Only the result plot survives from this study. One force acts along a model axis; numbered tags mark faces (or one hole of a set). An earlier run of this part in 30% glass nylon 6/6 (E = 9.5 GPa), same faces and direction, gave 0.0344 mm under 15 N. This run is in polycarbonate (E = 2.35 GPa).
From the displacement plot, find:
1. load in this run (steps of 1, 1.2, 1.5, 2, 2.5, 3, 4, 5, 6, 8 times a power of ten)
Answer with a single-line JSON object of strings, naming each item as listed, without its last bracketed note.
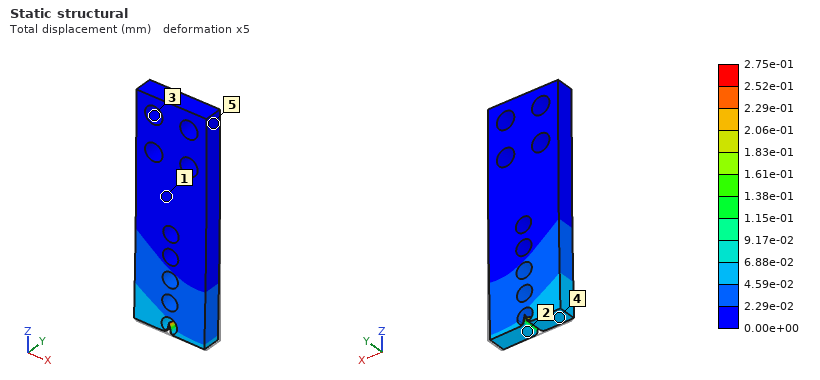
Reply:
{"load in this run": "30 N"}
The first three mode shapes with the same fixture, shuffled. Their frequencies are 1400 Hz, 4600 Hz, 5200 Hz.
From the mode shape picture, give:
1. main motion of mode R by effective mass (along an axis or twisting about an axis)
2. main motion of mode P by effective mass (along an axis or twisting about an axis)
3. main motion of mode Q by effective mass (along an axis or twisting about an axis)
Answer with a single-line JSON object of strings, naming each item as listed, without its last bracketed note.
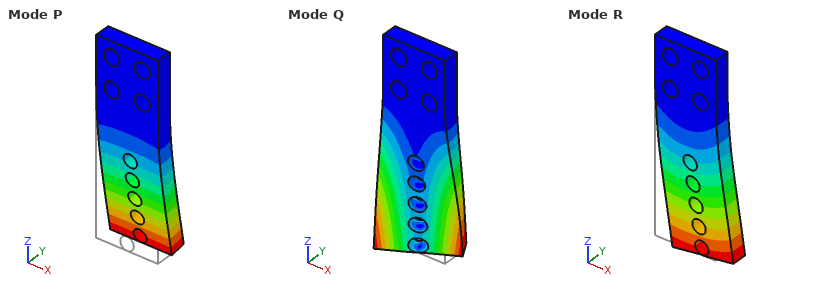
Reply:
{"main motion of mode R by effective mass": "along X", "main motion of mode P by effective mass": "along Y", "main motion of mode Q by effective mass": "twisting about Z"}
